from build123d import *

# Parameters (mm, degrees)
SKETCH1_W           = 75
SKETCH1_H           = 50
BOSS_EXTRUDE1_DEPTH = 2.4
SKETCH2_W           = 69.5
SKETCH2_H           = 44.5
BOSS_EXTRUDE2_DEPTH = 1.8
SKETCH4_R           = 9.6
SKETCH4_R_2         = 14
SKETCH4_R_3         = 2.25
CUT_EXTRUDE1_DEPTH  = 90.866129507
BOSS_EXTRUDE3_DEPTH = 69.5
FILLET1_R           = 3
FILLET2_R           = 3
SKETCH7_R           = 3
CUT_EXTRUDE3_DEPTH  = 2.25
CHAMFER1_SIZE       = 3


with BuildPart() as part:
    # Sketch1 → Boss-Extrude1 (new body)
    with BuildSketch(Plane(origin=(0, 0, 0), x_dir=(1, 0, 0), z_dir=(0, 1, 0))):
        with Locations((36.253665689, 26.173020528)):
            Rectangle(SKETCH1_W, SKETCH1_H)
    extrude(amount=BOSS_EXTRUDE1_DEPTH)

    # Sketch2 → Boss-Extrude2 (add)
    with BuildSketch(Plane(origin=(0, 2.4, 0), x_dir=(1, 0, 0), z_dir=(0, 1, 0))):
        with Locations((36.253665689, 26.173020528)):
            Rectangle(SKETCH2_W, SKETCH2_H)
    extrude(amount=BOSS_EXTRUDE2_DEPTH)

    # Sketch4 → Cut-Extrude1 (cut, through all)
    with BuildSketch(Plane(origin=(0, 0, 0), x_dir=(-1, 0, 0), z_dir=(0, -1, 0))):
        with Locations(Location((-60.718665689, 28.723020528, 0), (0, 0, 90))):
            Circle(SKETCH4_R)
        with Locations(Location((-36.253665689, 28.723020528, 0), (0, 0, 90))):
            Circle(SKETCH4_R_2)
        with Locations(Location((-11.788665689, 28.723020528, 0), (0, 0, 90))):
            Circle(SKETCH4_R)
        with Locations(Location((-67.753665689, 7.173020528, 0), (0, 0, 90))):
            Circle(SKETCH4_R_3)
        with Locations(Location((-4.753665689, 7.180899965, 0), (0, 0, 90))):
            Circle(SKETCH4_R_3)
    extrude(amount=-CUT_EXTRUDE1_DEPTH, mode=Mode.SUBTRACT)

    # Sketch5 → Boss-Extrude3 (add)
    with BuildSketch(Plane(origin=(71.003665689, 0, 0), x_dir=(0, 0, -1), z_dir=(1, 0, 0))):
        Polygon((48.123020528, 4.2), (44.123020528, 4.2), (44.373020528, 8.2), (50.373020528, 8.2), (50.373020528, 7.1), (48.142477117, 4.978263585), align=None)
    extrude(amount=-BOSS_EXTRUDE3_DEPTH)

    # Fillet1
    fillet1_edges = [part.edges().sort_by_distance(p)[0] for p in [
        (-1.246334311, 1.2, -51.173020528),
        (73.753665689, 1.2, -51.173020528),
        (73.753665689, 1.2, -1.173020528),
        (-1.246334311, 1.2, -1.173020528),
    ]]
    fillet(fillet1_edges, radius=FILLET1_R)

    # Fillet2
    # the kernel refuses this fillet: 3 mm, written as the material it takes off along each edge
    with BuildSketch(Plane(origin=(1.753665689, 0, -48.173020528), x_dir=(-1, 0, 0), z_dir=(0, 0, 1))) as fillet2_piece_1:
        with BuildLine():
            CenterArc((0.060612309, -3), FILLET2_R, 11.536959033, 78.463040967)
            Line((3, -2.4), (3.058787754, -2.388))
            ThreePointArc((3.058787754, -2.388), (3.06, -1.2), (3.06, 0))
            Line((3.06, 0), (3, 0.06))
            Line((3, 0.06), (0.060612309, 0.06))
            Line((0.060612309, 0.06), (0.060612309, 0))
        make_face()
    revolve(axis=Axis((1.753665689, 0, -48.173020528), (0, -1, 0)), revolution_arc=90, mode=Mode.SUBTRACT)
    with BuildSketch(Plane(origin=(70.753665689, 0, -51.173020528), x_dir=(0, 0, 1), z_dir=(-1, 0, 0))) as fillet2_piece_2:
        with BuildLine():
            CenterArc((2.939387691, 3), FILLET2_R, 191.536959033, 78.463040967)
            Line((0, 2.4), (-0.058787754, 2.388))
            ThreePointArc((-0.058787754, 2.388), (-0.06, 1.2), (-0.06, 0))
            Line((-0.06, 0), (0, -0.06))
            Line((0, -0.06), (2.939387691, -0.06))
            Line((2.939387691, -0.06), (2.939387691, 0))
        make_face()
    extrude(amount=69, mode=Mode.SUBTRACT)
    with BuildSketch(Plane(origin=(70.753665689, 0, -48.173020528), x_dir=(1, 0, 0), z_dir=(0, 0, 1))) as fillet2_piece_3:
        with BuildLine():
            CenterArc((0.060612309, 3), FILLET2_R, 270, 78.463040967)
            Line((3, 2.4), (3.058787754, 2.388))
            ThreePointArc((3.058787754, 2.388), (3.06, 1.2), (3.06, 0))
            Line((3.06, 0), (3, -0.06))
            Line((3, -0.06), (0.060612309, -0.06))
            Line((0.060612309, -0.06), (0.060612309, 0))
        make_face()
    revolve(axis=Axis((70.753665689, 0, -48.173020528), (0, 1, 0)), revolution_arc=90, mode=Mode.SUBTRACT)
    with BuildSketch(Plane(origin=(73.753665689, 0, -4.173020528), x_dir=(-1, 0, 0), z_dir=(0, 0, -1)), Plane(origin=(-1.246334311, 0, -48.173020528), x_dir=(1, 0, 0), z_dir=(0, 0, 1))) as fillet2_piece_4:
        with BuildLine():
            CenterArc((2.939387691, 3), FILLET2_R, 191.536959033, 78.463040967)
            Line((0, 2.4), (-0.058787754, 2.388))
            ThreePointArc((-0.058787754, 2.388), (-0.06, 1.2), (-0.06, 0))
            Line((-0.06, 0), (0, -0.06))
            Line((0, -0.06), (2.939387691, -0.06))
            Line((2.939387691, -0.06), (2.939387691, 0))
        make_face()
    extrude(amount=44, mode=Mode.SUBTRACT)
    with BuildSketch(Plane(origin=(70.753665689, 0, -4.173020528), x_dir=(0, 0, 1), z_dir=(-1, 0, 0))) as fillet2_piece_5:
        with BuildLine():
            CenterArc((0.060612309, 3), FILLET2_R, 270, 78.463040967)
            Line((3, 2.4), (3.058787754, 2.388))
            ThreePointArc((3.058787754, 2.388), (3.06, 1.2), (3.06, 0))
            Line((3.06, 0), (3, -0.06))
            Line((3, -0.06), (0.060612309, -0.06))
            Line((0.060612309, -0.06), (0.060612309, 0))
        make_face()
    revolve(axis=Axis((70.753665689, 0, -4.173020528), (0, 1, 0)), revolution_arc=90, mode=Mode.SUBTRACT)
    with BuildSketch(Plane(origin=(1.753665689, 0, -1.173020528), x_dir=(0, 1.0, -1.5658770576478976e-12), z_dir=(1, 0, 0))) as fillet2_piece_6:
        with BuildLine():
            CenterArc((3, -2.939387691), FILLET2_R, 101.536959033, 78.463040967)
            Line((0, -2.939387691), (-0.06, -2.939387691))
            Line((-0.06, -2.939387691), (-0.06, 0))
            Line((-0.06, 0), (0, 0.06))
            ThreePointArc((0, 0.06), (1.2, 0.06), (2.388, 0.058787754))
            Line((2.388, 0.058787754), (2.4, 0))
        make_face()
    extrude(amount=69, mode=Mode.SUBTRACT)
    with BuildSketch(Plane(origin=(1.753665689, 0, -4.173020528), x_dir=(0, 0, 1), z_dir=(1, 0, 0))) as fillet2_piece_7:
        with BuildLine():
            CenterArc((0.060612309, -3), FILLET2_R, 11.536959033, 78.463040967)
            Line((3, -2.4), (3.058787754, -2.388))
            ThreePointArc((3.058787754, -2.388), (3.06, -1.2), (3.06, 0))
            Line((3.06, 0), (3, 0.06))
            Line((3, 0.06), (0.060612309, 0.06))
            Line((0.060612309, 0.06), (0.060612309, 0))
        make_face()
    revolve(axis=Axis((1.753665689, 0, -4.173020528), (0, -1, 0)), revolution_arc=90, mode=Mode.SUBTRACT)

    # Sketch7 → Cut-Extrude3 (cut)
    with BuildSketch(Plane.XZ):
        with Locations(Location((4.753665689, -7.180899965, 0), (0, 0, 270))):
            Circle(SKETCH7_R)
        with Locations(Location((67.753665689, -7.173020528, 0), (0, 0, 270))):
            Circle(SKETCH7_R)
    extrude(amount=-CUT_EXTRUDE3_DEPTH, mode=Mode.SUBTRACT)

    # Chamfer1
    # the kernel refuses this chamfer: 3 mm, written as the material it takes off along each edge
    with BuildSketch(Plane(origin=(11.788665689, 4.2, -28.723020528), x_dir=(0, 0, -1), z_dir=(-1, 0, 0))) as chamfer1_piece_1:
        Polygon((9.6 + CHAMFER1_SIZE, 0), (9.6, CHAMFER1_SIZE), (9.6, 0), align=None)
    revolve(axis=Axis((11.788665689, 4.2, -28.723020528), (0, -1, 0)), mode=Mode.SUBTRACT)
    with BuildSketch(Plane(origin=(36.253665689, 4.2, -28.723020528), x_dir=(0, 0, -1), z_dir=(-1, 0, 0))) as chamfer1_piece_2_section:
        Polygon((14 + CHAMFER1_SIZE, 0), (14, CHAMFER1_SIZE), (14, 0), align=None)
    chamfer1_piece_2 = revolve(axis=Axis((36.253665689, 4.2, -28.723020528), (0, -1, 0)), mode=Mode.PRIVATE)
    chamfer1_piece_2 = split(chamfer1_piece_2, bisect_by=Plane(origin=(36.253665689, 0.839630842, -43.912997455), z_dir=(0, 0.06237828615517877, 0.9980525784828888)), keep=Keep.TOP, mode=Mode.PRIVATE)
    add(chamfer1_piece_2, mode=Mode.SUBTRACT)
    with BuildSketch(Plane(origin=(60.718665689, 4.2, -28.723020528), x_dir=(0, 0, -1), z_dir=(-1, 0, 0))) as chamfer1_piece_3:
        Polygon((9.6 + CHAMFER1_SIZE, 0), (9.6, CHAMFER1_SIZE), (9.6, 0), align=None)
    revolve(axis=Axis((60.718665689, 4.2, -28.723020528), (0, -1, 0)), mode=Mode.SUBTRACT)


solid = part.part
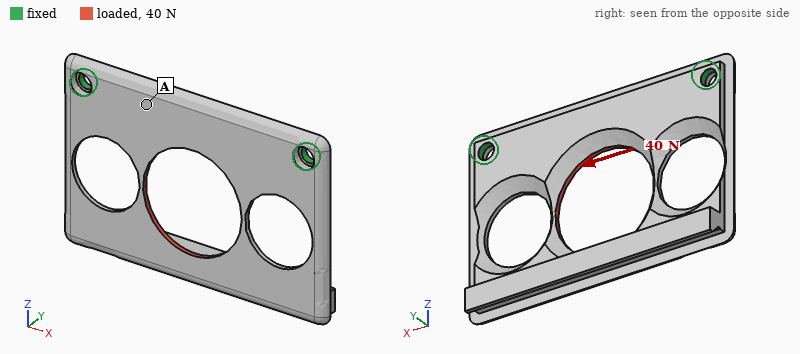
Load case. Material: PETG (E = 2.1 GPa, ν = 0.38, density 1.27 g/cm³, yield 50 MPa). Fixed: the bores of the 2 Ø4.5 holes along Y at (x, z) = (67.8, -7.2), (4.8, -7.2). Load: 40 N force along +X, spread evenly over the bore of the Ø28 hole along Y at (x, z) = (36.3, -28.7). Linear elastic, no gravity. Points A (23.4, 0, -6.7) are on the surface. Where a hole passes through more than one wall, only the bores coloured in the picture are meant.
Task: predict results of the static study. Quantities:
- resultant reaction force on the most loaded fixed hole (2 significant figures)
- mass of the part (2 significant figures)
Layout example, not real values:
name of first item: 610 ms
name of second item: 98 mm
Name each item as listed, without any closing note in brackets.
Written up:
resultant reaction force on the most loaded fixed hole: 24 N
mass of the part: 12 g
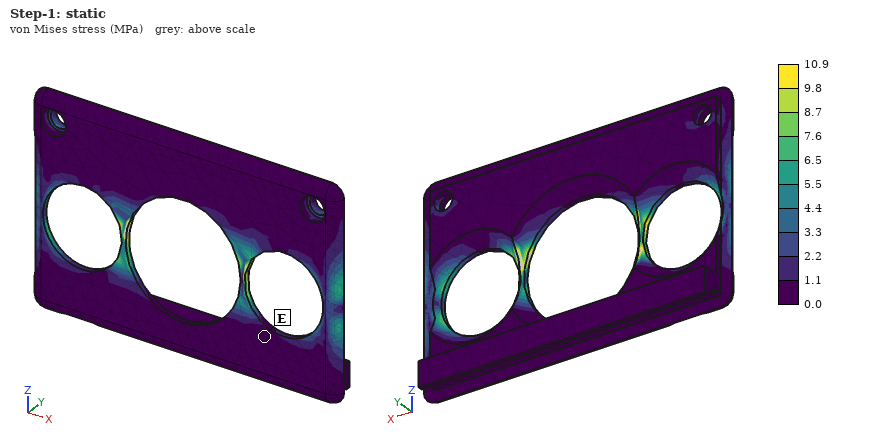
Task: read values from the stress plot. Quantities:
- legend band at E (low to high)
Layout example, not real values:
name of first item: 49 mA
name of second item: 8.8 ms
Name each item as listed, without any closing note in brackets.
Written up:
legend band at E: 0.0 to 1.1 MPa
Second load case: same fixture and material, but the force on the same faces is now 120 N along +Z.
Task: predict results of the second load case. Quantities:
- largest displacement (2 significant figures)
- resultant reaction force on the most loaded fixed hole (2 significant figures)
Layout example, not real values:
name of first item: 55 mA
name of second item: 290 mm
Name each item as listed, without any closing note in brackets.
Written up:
largest displacement: 0.90 mm
resultant reaction force on the most loaded fixed hole: 64 N
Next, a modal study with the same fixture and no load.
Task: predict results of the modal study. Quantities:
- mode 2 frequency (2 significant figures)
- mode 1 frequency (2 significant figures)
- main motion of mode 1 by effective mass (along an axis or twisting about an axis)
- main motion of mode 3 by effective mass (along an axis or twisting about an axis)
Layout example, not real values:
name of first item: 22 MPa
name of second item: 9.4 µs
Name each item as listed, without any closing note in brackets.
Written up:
mode 2 frequency: 420 Hz
mode 1 frequency: 110 Hz
main motion of mode 1 by effective mass: along Y
main motion of mode 3 by effective mass: along X
